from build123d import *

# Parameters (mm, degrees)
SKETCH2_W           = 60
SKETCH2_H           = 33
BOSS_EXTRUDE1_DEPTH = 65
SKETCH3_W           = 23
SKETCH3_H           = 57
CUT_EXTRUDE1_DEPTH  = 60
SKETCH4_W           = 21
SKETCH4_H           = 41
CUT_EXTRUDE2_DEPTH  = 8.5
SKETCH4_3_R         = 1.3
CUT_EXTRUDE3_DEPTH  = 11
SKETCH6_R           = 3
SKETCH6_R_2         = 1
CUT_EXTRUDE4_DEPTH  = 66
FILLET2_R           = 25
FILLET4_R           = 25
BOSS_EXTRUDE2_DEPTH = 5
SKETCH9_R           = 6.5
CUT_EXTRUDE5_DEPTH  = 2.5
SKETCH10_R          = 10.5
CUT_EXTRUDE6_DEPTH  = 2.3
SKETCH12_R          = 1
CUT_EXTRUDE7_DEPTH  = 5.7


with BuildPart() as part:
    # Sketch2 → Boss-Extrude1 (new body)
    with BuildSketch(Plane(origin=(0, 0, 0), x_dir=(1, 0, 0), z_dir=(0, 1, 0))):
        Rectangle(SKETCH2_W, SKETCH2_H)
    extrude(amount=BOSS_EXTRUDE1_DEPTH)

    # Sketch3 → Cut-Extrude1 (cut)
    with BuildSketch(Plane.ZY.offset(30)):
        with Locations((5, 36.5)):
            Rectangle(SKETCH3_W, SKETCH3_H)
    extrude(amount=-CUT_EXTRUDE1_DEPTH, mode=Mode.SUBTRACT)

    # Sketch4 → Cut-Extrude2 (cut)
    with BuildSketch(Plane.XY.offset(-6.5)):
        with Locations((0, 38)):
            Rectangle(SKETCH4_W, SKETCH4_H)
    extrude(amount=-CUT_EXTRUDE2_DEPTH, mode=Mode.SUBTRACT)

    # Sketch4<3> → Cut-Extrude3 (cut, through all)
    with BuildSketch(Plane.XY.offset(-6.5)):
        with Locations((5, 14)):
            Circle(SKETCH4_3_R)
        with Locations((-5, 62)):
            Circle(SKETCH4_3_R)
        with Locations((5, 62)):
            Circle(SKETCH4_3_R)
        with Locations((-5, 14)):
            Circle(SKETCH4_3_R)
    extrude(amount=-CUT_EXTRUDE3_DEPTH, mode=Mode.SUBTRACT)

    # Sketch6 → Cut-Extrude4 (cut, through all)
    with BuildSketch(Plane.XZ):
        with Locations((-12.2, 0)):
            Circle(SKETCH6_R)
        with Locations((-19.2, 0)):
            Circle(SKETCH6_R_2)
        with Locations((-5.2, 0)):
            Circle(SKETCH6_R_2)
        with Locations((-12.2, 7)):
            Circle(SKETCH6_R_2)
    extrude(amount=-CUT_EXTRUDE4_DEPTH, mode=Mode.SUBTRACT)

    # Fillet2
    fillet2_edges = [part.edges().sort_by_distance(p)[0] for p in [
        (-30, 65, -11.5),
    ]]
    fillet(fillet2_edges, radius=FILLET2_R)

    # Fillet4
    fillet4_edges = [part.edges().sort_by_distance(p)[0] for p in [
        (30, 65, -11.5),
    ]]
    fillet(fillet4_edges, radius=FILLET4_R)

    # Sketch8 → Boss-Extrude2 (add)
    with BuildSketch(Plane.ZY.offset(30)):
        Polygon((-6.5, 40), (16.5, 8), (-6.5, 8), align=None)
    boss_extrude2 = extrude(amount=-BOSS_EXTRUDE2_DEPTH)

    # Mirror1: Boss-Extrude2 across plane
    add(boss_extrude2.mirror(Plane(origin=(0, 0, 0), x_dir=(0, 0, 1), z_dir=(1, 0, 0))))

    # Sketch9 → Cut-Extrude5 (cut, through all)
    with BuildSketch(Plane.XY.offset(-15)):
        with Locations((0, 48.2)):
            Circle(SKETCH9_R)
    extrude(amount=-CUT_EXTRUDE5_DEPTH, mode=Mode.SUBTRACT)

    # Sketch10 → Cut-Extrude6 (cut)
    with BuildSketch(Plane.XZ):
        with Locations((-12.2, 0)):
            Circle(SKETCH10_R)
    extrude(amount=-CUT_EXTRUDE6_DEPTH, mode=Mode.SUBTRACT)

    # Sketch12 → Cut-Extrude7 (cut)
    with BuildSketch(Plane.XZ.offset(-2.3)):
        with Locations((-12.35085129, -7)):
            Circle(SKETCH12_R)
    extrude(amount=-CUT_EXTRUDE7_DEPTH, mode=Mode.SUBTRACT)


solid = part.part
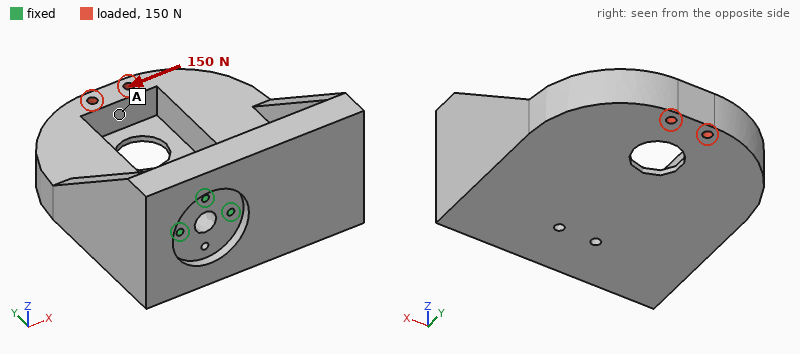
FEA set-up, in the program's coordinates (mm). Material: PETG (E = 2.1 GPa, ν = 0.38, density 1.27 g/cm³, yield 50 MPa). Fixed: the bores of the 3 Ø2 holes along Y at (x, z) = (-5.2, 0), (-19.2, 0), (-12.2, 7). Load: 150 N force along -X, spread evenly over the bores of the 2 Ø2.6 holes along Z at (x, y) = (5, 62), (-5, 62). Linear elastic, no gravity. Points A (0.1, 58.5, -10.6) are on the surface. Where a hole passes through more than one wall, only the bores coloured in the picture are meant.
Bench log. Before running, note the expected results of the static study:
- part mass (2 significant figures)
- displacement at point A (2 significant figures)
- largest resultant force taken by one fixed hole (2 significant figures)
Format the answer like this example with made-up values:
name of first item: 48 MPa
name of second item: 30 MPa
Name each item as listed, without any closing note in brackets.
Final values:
part mass: 54 g
displacement at point A: 0.96 mm
largest resultant force taken by one fixed hole: 440 N
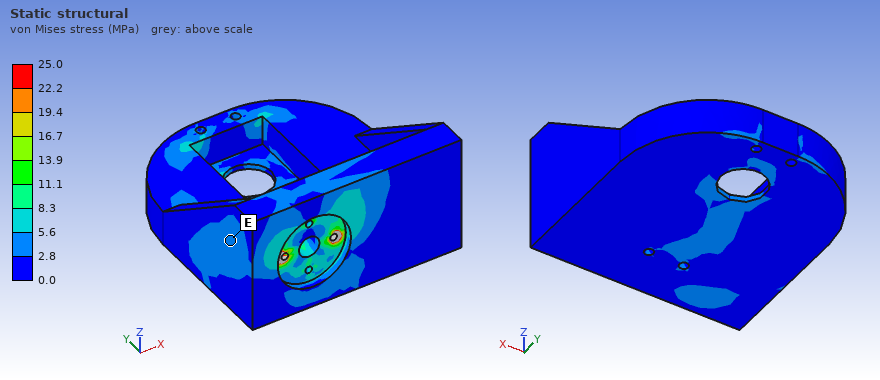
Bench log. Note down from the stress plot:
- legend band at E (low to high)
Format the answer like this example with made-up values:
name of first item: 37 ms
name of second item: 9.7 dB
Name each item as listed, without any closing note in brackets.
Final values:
legend band at E: 2.8 to 5.6 MPa
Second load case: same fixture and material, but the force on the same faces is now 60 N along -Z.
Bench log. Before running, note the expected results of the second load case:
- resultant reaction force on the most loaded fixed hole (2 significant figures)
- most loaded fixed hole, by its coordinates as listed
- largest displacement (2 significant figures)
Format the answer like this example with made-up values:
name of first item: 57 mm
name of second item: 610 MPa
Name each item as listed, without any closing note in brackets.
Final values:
resultant reaction force on the most loaded fixed hole: 170 N
most loaded fixed hole, by its coordinates as listed: (-12.2, 7)
largest displacement: 1.1 mm
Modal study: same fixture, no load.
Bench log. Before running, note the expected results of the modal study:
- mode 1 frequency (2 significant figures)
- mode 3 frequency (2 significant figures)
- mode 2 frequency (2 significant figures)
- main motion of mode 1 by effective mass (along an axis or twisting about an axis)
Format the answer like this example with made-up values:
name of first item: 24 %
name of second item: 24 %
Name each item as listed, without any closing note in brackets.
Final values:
mode 1 frequency: 390 Hz
mode 3 frequency: 980 Hz
mode 2 frequency: 480 Hz
main motion of mode 1 by effective mass: along Z
